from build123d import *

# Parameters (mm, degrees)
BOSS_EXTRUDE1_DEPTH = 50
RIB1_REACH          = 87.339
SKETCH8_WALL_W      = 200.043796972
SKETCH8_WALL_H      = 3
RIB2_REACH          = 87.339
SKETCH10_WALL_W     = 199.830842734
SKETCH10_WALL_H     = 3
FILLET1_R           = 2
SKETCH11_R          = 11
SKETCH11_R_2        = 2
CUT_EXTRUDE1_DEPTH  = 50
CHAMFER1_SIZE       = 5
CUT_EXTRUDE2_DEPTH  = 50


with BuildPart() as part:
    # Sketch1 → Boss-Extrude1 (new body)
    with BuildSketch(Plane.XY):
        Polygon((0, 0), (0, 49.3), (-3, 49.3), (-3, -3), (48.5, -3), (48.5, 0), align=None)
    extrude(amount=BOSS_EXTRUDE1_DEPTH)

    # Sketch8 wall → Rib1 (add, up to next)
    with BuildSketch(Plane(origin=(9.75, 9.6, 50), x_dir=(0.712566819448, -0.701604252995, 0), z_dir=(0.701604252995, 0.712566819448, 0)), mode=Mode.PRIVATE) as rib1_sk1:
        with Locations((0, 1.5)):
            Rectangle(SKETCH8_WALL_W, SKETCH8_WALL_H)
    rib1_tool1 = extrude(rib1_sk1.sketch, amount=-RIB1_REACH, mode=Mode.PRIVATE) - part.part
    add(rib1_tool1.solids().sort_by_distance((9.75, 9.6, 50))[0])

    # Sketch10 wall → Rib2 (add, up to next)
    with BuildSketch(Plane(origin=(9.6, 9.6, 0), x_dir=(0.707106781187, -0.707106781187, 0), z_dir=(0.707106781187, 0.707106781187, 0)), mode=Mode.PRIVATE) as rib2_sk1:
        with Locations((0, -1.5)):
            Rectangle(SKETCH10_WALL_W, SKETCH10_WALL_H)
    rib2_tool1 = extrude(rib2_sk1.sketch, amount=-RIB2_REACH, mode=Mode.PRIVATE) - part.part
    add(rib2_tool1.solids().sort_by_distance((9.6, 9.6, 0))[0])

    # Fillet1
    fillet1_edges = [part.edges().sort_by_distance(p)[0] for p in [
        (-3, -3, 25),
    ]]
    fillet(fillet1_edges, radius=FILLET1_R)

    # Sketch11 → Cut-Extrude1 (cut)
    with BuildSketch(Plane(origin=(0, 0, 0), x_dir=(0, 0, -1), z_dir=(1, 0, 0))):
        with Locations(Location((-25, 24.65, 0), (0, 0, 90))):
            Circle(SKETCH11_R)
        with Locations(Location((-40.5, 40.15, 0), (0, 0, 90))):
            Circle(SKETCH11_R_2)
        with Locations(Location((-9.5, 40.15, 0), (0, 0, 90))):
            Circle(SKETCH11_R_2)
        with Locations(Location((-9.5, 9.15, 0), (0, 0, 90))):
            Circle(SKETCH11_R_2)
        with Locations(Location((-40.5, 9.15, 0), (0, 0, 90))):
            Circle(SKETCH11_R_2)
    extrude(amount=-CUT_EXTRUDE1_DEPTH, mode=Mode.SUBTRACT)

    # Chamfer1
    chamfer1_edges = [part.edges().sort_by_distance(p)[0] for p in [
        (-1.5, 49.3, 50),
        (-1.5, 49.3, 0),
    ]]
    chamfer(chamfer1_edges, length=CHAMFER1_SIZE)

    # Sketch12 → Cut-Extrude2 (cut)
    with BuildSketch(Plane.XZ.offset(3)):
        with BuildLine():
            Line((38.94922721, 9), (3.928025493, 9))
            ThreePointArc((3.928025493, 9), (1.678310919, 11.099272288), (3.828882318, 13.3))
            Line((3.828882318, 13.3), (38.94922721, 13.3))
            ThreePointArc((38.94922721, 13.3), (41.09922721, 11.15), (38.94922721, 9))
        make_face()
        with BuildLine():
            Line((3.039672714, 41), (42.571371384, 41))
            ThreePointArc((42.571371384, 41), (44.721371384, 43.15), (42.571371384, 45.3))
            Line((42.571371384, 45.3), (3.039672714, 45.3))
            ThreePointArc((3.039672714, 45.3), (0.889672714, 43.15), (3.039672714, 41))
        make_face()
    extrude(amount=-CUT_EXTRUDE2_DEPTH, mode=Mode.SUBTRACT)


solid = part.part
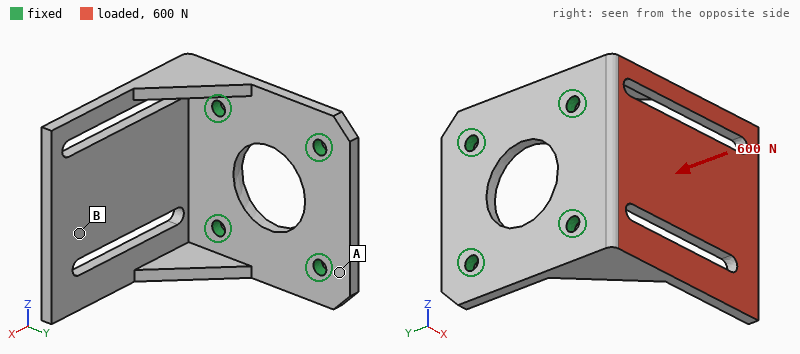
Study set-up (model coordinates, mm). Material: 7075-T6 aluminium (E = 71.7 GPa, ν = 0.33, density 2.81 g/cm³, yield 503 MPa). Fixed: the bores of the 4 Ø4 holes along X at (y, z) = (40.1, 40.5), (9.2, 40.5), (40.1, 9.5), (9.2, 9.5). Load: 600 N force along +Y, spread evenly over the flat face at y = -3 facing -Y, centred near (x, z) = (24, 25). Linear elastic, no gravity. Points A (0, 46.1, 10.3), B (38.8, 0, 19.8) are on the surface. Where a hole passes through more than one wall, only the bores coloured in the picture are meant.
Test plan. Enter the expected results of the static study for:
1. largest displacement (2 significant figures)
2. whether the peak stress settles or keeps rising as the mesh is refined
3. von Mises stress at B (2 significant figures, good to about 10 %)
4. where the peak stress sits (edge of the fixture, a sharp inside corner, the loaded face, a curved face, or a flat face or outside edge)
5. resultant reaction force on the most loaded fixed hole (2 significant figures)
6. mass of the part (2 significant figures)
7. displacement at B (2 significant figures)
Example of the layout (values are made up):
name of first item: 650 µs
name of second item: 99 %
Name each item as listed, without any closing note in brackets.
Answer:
largest displacement: 1.0 mm
whether the peak stress settles or keeps rising as the mesh is refined: keeps rising
von Mises stress at B: 40 MPa
where the peak stress sits: edge of the fixture
resultant reaction force on the most loaded fixed hole: 290 N
mass of the part: 39 g
displacement at B: 0.74 mm
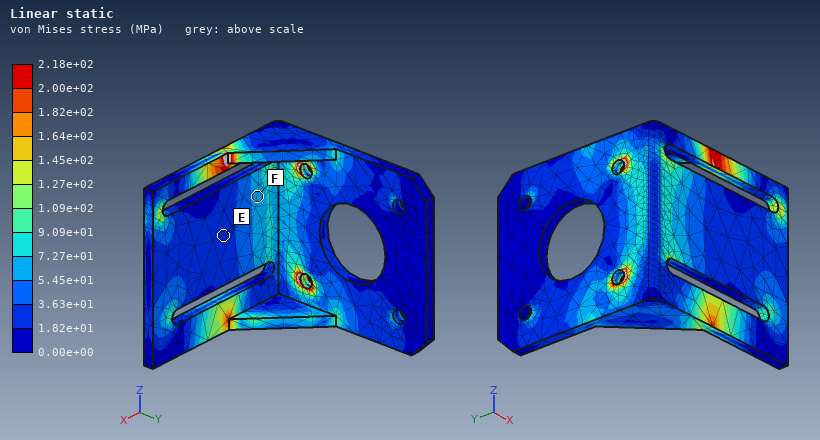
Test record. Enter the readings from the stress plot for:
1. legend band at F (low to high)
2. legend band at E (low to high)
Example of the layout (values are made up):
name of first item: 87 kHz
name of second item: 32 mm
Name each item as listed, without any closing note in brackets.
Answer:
legend band at F: 5.45e+01 to 7.27e+01 MPa
legend band at E: 1.82e+01 to 3.63e+01 MPa
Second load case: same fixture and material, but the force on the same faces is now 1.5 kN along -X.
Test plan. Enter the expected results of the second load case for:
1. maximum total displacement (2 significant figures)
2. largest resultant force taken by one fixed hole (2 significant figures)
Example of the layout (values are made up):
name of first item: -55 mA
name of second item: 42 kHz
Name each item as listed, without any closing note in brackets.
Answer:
maximum total displacement: 0.47 mm
largest resultant force taken by one fixed hole: 890 N
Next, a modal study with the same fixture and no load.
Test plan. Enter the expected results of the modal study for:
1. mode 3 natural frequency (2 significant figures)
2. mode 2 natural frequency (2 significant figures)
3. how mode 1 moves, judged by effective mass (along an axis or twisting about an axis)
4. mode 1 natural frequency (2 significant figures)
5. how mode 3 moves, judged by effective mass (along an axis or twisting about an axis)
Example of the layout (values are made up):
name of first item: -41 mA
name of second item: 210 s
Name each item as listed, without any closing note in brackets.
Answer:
mode 3 natural frequency: 3800 Hz
mode 2 natural frequency: 2600 Hz
how mode 1 moves, judged by effective mass: along Y
mode 1 natural frequency: 1100 Hz
how mode 3 moves, judged by effective mass: along Z
